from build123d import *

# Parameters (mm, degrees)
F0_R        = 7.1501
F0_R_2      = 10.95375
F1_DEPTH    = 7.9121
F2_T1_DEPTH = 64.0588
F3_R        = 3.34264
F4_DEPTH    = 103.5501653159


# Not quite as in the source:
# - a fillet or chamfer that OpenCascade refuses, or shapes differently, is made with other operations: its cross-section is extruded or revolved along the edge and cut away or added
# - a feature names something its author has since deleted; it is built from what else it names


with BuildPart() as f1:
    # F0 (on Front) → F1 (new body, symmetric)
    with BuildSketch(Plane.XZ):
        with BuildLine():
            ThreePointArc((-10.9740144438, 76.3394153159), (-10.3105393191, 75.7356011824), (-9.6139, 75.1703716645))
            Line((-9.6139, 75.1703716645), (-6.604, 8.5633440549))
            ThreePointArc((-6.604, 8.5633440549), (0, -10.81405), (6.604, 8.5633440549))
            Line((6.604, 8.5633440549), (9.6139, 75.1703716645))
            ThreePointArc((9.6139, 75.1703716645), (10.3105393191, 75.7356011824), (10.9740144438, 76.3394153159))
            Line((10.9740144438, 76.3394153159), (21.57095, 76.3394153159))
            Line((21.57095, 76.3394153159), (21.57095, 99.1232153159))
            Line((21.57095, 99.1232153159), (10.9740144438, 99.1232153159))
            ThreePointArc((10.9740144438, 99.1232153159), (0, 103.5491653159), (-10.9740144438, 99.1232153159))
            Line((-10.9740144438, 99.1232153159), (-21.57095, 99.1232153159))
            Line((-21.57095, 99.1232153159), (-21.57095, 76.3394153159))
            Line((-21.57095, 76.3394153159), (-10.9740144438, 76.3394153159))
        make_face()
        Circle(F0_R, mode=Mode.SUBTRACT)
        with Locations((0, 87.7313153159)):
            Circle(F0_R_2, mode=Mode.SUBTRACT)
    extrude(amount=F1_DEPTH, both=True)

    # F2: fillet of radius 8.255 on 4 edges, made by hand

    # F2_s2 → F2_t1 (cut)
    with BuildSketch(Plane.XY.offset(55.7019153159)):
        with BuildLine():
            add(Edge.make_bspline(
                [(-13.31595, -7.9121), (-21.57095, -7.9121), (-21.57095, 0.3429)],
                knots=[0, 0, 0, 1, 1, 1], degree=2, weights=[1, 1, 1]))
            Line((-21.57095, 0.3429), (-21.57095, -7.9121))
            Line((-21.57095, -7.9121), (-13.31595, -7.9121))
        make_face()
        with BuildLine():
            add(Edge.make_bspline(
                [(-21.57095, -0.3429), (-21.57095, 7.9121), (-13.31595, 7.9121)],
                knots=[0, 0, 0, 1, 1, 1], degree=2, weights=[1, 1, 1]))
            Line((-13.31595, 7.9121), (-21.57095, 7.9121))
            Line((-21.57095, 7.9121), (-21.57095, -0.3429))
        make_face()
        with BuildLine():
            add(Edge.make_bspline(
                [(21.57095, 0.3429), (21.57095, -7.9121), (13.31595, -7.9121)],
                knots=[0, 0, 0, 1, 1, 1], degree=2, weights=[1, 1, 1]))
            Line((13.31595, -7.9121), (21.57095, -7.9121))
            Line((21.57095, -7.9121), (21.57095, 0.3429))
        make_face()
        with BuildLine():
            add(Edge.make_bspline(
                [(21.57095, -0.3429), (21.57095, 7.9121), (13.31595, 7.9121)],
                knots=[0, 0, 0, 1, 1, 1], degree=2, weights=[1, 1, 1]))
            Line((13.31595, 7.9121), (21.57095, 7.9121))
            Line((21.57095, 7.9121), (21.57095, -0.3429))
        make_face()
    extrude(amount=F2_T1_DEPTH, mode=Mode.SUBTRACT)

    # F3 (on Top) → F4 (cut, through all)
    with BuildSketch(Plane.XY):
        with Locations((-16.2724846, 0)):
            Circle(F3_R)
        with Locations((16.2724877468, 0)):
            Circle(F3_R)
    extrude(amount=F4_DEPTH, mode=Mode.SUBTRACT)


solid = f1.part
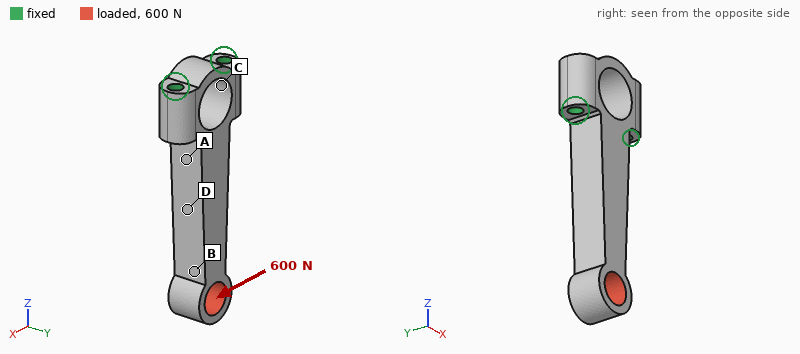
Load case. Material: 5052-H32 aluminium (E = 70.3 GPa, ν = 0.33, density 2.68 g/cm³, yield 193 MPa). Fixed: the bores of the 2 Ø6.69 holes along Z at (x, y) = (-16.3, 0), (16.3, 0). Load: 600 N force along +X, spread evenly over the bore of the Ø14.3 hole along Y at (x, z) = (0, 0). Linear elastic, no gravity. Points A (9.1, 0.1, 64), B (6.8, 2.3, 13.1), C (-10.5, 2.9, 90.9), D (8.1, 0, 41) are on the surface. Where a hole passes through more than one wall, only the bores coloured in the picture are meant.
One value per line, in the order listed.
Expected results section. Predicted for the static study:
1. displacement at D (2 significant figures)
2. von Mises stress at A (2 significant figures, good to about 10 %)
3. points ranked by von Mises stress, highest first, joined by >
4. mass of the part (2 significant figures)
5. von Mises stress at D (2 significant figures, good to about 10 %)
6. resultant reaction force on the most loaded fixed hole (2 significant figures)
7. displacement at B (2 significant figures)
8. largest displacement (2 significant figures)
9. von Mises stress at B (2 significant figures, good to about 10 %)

0.078 mm
45 MPa
A > D > B > C
76 g
36 MPa
2.4 kN
0.19 mm
0.33 mm
18 MPa
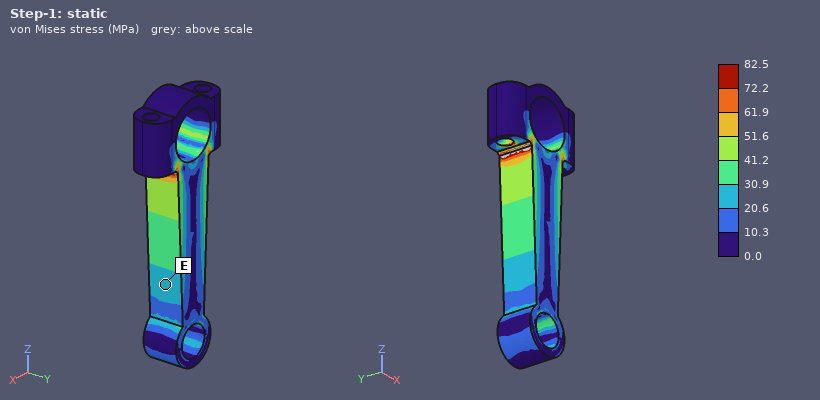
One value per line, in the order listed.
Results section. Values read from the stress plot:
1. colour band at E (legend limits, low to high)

20.6 to 30.9 MPa
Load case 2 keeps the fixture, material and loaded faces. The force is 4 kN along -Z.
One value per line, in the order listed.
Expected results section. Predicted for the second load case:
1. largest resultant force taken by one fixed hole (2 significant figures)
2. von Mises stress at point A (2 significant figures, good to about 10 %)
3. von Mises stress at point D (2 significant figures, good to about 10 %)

2.3 kN
14 MPa
16 MPa
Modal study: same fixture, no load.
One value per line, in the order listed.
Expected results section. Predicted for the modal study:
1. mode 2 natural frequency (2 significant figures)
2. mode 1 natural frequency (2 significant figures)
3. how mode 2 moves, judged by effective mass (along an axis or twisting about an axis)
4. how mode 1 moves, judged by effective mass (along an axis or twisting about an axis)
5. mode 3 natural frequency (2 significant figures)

1900 Hz
1300 Hz
along X
along Y
7600 Hz
